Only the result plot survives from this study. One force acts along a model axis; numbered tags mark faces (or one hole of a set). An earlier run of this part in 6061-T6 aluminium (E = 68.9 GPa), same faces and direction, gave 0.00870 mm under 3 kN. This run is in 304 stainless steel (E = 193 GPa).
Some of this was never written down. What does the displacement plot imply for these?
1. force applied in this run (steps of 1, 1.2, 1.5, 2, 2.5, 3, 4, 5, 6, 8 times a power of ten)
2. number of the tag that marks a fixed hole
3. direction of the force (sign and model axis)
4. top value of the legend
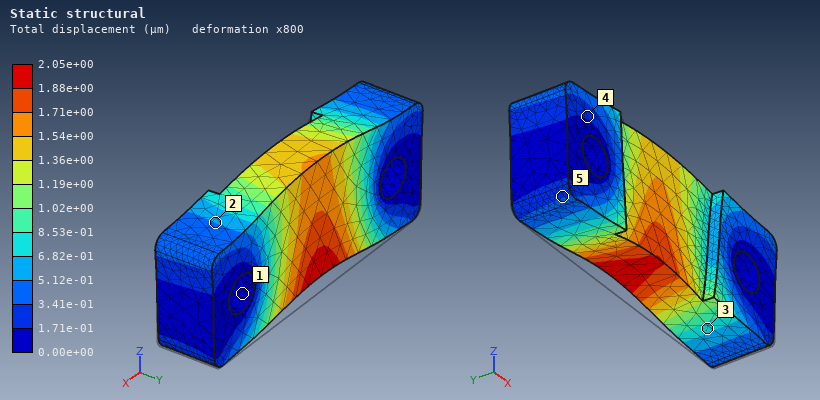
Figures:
2 kN
1
+Z
2.05e+00 µm
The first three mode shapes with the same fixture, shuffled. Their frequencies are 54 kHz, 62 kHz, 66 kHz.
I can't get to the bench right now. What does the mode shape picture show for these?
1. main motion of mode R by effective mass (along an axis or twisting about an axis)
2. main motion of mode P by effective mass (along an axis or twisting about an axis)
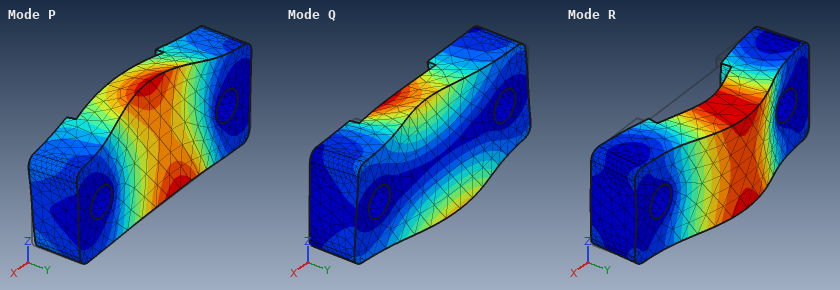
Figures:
along Y
along Z
